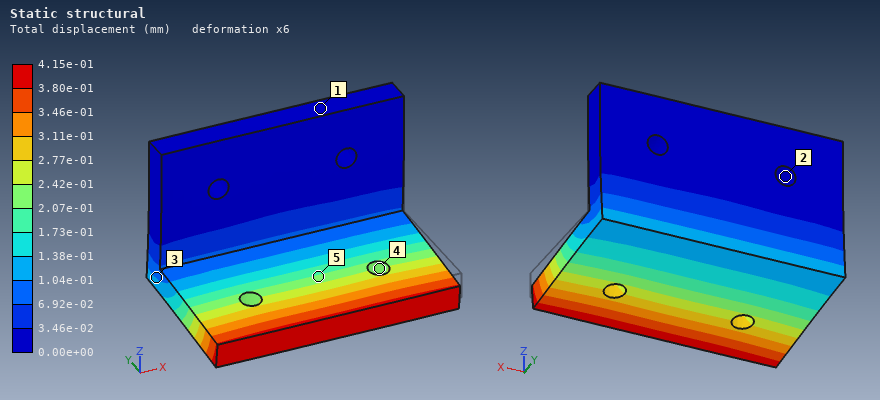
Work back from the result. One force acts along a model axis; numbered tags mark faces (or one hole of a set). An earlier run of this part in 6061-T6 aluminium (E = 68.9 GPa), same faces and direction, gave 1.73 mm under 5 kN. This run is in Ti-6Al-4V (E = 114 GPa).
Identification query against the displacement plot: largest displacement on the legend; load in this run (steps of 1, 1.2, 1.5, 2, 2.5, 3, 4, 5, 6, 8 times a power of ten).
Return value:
4.15e-01 mm
2 kN
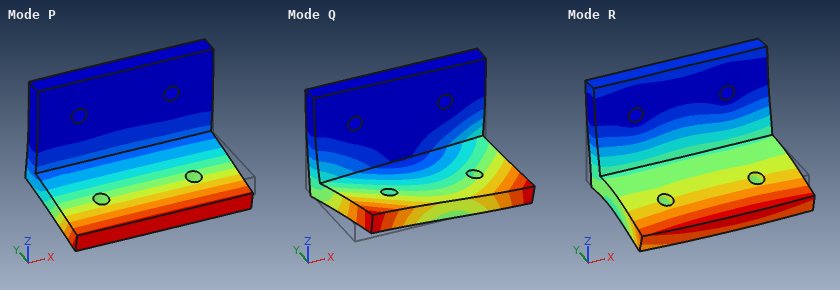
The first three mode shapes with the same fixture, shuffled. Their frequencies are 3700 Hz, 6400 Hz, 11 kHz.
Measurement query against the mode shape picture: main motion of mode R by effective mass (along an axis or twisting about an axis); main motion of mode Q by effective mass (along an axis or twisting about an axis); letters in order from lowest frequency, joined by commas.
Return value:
along Y
along X
P, Q, R
